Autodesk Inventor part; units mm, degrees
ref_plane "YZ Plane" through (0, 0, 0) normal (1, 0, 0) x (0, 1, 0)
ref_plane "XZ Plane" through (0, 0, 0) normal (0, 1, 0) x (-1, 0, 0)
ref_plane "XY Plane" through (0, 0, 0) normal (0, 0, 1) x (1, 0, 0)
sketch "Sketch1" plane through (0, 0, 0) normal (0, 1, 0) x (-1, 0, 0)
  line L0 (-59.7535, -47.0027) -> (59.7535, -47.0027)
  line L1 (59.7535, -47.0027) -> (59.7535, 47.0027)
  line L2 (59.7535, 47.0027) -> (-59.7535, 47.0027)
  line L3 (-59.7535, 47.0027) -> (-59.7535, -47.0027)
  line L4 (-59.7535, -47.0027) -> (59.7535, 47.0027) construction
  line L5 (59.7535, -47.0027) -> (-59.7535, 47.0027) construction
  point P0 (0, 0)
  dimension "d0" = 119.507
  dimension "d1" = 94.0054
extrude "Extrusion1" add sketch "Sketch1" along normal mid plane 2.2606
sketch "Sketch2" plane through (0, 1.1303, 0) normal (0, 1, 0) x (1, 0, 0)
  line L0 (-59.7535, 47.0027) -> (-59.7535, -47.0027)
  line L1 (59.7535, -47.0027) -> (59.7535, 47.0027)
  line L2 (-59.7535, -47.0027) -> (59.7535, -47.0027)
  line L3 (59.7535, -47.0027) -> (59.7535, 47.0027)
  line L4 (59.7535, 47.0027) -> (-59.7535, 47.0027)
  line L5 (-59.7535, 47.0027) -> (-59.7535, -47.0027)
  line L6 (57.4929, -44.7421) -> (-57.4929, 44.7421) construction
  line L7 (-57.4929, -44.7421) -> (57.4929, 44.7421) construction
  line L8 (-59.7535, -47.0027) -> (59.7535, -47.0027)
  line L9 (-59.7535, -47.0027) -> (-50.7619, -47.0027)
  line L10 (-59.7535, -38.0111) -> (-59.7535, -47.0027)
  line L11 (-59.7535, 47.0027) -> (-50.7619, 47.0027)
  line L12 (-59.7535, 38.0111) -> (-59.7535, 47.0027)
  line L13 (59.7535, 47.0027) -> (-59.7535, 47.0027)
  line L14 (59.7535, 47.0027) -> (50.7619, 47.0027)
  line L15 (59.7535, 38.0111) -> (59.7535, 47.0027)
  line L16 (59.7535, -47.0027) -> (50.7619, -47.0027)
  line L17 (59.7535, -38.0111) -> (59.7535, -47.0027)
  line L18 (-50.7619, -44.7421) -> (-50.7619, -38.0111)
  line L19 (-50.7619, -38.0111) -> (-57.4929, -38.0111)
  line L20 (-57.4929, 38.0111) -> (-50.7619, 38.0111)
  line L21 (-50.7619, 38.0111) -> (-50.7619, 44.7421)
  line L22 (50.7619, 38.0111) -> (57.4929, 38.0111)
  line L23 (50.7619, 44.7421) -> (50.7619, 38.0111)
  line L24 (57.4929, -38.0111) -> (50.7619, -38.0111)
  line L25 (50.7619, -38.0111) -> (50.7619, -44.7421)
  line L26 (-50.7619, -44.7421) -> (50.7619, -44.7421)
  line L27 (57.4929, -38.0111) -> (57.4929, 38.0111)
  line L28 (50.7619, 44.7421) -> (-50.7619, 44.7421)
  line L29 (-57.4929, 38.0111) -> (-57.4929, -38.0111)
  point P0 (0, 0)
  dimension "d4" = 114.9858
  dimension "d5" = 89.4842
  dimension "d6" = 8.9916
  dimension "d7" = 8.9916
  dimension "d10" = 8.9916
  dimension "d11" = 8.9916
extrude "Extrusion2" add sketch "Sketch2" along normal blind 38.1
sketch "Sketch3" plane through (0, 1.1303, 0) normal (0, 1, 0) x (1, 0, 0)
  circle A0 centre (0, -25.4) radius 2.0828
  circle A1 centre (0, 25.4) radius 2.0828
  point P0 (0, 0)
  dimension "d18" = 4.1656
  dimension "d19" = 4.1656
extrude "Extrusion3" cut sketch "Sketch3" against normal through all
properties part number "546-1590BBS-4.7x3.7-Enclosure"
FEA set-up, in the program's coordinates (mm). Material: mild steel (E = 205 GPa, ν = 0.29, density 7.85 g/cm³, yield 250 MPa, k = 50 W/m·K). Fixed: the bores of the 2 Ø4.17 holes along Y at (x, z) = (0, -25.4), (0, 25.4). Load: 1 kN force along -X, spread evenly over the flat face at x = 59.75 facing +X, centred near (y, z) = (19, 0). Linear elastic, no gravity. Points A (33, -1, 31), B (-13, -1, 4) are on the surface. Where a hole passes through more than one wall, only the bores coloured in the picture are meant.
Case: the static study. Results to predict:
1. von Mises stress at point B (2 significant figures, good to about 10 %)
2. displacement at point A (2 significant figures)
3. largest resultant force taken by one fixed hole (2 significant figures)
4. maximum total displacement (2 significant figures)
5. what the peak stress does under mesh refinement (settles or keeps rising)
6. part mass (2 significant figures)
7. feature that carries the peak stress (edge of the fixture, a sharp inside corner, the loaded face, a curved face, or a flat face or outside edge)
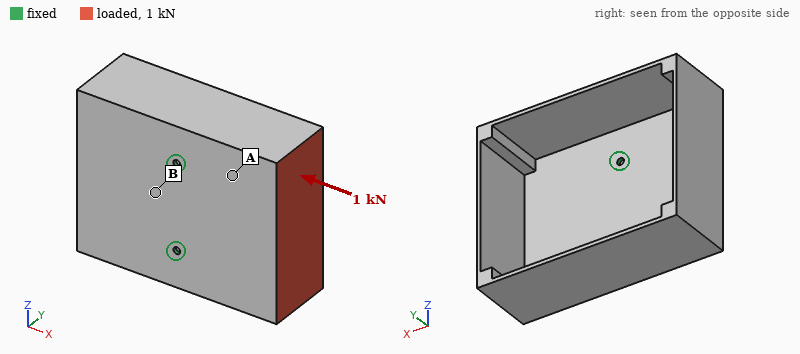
49 MPa
0.26 mm
500 N
0.70 mm
keeps rising
540 g
edge of the fixture
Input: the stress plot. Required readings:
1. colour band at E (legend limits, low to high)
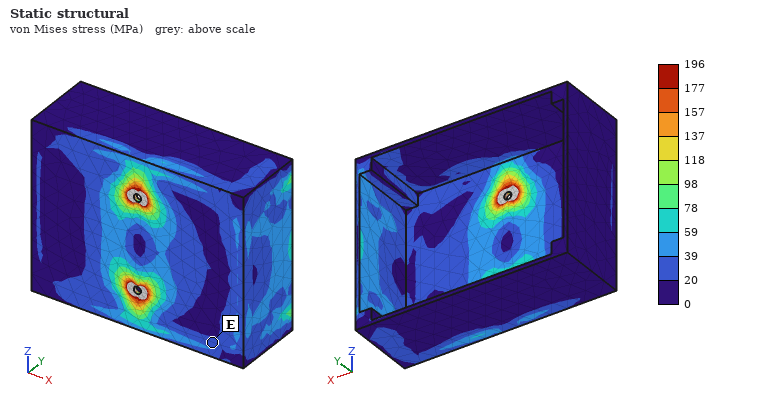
20 to 39 MPa
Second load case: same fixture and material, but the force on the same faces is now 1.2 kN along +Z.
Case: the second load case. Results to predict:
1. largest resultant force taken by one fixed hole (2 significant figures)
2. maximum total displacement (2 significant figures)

1.5 kN
0.44 mm
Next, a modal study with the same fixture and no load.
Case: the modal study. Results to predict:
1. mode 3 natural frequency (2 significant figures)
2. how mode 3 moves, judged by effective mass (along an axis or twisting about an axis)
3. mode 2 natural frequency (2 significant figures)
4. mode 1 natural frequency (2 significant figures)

670 Hz
along Z
450 Hz
220 Hz
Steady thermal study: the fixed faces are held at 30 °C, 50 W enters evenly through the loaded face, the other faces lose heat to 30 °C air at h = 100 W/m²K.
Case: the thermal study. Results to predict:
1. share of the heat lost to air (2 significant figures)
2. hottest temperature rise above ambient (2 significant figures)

96 %
64 K
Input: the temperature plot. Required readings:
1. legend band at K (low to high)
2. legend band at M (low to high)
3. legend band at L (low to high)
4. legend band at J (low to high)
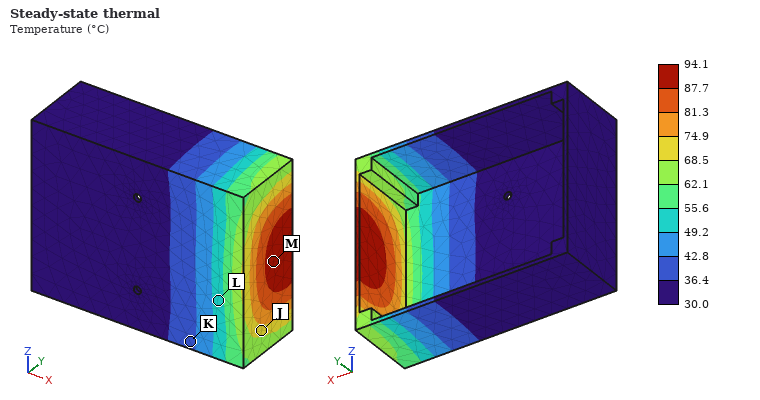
36.4 to 42.8 °C
87.7 to 94.1 °C
49.2 to 55.6 °C
68.5 to 74.9 °C
